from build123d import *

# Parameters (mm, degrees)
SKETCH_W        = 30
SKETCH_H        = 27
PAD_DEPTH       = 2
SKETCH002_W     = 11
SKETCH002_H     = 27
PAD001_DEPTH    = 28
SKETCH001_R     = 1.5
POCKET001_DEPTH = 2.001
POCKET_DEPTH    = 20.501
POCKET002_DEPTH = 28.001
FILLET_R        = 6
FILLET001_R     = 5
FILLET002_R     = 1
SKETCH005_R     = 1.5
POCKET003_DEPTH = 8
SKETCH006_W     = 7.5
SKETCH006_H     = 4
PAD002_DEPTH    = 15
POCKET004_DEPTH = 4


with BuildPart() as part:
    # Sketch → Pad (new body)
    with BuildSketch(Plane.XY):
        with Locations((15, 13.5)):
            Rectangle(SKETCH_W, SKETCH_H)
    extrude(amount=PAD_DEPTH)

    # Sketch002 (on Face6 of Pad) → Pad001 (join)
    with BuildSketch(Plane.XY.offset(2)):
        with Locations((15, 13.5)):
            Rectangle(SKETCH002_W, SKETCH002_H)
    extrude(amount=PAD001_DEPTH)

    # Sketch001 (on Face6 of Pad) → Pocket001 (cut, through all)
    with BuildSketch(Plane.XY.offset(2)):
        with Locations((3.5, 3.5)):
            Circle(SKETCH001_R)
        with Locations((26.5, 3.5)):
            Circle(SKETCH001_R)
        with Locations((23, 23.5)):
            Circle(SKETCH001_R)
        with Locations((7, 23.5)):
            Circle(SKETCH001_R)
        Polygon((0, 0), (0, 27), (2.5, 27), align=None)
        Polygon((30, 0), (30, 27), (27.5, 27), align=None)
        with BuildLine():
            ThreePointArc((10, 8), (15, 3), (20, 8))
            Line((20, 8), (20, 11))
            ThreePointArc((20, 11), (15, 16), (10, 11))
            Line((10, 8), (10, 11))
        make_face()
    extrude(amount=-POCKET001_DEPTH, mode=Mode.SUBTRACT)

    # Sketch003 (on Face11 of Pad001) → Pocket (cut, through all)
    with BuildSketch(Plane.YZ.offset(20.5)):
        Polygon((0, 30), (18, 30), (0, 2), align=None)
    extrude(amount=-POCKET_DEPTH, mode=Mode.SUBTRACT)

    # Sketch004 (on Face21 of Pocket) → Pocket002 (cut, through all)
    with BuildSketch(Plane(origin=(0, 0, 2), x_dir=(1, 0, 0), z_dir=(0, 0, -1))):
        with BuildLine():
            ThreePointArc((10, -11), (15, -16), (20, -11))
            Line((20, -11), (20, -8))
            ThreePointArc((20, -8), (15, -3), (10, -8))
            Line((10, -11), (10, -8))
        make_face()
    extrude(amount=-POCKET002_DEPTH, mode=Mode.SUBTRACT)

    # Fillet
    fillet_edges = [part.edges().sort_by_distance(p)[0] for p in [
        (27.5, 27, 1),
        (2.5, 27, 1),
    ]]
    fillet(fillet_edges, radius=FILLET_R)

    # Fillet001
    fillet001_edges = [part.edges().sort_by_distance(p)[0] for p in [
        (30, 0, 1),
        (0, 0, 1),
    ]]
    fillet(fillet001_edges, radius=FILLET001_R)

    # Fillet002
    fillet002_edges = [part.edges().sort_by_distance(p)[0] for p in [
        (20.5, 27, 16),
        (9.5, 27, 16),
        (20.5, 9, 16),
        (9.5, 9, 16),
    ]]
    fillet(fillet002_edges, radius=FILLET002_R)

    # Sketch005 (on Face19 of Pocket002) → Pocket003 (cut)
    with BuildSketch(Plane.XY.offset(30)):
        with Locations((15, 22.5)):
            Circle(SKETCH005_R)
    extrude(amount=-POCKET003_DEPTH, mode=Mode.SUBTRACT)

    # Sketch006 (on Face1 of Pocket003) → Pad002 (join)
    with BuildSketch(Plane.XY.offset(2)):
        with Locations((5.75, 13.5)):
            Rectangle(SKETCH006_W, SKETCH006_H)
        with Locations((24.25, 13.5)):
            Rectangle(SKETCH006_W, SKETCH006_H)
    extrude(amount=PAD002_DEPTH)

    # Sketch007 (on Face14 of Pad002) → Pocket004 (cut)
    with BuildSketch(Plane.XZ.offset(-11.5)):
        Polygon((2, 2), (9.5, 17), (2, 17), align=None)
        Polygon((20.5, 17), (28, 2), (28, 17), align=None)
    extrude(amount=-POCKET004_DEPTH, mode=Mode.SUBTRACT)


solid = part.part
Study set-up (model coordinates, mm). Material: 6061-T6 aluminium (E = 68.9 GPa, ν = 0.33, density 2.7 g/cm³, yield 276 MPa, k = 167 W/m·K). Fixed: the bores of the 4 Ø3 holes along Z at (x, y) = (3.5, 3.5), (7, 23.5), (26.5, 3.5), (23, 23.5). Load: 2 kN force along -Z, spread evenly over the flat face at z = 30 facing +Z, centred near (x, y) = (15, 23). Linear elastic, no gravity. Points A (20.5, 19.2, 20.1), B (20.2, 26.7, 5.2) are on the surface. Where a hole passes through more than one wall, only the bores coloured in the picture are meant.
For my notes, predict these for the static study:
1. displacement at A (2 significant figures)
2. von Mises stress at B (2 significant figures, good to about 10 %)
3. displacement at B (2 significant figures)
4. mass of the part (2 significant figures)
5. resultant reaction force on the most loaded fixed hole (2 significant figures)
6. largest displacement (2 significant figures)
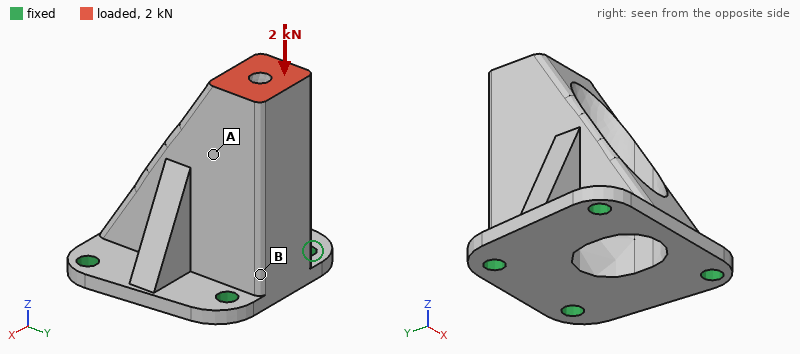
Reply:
17 µm
39 MPa
14 µm
15 g
1.0 kN
33 µm
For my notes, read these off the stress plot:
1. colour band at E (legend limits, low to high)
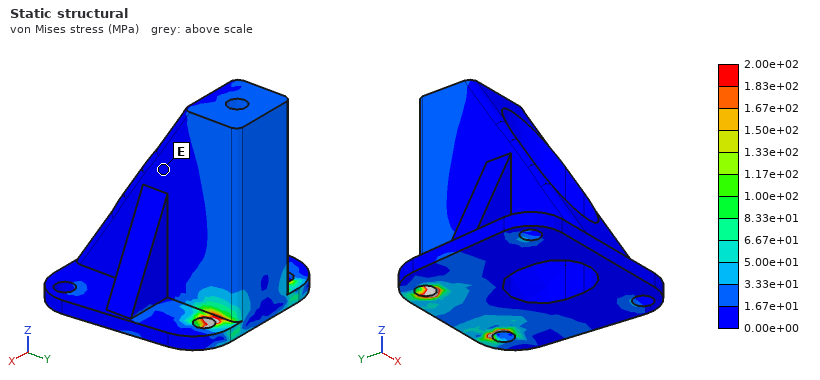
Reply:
0.00e+00 to 1.67e+01 MPa
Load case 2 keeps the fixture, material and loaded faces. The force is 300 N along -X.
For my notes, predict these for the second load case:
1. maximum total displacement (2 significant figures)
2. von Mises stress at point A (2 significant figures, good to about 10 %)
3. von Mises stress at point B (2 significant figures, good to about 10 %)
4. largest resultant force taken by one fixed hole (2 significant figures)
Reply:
44 µm
11 MPa
23 MPa
490 N
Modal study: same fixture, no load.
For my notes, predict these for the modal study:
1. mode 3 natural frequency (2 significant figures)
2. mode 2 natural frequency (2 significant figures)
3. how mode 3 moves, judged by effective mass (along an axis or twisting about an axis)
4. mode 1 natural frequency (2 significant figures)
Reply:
18 kHz
7800 Hz
along Z
7600 Hz
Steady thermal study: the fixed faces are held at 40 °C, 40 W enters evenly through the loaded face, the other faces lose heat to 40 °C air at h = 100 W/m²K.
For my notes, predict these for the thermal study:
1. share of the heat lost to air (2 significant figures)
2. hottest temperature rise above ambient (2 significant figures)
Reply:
16 %
60 K
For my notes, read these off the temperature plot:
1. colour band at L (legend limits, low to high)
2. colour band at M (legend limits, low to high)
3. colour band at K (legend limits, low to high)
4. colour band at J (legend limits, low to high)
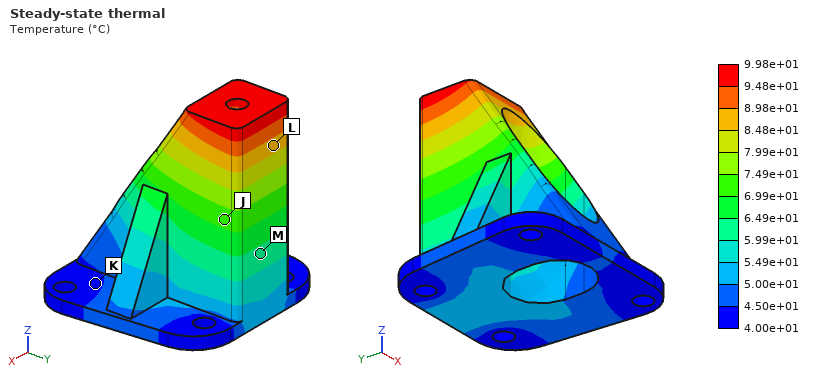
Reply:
8.48e+01 to 8.98e+01 °C
5.99e+01 to 6.49e+01 °C
4.00e+01 to 4.50e+01 °C
6.99e+01 to 7.49e+01 °C
